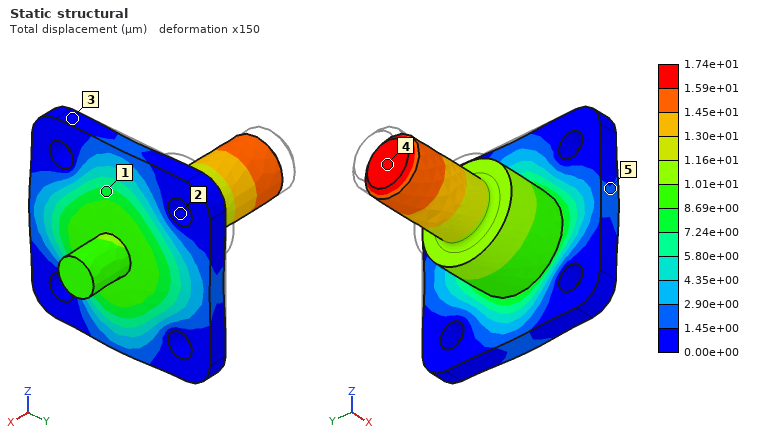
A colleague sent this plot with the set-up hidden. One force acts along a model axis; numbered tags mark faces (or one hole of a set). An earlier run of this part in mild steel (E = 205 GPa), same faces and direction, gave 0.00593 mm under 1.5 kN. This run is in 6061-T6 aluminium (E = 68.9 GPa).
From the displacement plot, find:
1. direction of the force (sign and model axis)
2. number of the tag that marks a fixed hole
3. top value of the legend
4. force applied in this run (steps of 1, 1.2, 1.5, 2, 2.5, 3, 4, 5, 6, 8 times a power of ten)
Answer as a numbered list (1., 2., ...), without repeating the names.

1. +X
2. 2
3. 1.74e+01 µm
4. 1.5 kN
